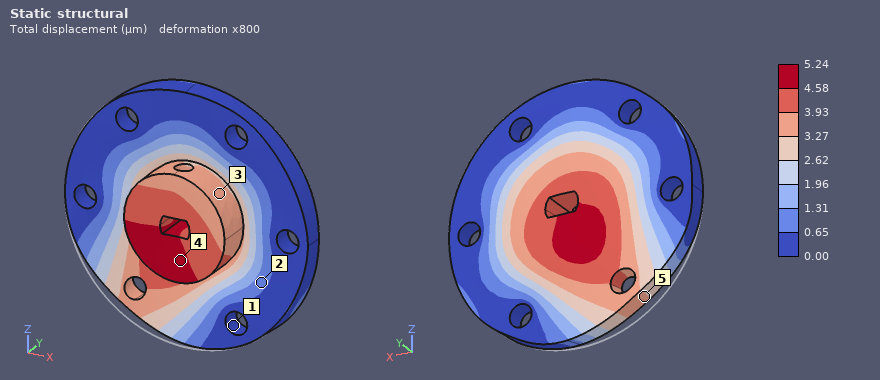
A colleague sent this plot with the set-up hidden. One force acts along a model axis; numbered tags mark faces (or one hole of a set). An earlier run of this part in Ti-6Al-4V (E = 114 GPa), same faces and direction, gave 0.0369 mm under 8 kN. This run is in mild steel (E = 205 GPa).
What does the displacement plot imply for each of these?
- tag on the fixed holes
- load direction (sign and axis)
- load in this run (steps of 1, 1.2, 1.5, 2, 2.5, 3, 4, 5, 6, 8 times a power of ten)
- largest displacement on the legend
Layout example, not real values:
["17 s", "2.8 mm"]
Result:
["1", "+Y", "2 kN", "5.24 µm"]
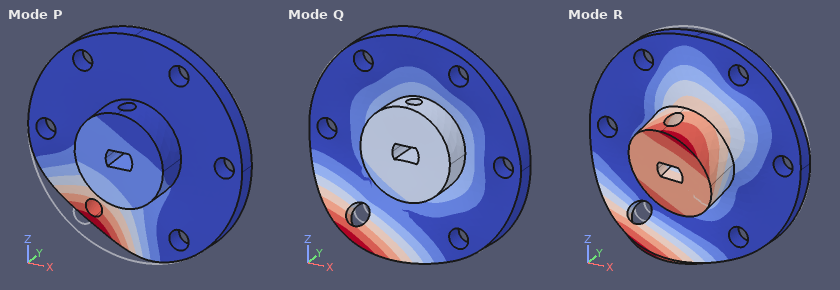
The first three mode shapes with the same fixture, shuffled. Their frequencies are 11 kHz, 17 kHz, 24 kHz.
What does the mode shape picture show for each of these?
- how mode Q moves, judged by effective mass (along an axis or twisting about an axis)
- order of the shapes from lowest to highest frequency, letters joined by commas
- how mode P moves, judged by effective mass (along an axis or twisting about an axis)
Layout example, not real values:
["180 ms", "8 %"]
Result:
["along Y", "P, Q, R", "along Y"]
